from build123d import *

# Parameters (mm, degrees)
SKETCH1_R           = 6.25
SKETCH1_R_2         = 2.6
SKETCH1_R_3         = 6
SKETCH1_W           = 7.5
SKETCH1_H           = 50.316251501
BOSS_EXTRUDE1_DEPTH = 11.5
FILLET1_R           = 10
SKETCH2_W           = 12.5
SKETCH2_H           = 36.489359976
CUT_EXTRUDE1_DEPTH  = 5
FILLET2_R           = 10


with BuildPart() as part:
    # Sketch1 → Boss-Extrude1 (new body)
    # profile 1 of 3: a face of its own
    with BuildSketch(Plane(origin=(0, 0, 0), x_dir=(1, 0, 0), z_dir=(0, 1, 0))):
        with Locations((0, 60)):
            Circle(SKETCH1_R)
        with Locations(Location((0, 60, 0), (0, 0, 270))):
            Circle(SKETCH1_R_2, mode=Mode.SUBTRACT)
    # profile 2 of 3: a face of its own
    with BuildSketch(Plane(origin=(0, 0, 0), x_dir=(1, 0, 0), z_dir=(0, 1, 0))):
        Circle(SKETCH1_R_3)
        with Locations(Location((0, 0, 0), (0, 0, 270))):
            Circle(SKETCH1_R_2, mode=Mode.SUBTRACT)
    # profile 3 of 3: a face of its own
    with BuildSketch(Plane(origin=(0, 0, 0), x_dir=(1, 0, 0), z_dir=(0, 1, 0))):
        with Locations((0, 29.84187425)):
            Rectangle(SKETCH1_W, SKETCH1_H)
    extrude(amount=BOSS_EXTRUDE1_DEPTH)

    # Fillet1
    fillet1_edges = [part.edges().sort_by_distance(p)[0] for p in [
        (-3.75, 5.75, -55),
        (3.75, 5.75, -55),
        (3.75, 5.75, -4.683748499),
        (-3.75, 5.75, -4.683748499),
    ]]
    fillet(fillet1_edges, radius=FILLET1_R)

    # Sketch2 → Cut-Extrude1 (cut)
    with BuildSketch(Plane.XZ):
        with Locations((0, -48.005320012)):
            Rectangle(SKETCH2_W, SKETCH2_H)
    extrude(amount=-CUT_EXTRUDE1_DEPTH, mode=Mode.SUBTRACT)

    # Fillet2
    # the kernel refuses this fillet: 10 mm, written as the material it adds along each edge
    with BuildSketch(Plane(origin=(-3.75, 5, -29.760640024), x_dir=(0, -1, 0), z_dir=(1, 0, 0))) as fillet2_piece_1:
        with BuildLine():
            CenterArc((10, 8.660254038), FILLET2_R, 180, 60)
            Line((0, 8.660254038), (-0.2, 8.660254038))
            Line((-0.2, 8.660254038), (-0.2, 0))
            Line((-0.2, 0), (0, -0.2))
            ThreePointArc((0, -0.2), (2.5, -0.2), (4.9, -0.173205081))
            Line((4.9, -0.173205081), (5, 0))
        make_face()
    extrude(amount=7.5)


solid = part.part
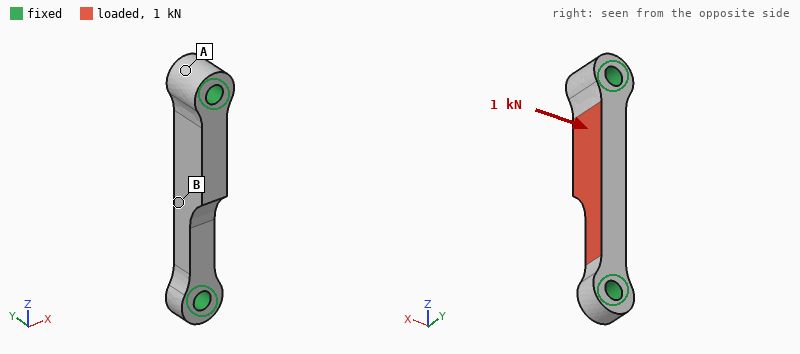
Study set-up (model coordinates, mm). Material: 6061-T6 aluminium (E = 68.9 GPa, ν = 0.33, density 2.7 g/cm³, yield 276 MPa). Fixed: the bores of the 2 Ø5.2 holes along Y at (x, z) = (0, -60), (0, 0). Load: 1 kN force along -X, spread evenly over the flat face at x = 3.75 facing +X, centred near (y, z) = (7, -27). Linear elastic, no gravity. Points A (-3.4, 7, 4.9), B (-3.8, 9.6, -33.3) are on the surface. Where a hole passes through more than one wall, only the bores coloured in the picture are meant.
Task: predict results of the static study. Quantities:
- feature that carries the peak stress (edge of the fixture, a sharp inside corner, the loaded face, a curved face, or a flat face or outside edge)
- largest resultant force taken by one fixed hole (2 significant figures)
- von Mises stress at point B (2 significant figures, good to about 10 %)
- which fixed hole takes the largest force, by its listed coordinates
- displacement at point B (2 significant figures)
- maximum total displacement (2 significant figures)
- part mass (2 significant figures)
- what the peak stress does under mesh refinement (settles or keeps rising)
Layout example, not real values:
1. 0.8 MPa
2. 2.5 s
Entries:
1. edge of the fixture
2. 600 N
3. 37 MPa
4. (0, 0)
5. 30 µm
6. 33 µm
7. 14 g
8. keeps rising
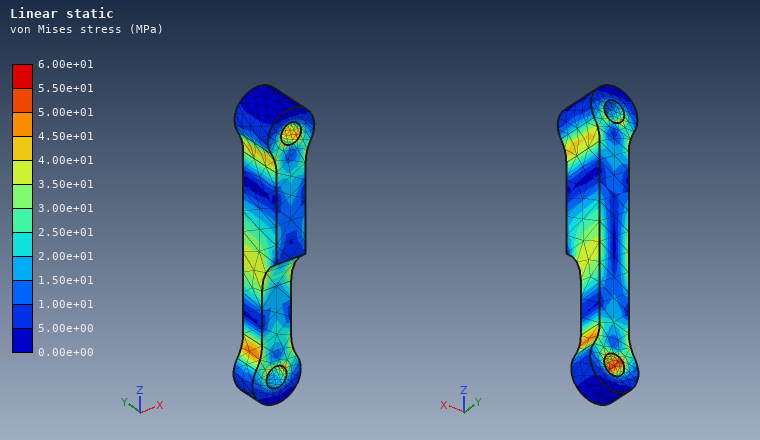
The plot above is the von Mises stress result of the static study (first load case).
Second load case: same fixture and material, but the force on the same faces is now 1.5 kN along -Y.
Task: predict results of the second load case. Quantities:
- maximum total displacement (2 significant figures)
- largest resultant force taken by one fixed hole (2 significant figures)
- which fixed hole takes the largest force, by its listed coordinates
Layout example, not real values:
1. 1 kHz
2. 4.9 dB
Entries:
1. 52 µm
2. 990 N
3. (0, 0)
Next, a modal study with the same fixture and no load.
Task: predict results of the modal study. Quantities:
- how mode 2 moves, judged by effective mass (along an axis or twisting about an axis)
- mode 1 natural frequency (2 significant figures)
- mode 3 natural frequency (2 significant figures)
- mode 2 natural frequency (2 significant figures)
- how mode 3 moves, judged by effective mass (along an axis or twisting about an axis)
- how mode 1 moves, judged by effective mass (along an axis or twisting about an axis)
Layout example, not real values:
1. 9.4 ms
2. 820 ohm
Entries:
1. along Y
2. 11 kHz
3. 24 kHz
4. 12 kHz
5. twisting about Z
6. along X
